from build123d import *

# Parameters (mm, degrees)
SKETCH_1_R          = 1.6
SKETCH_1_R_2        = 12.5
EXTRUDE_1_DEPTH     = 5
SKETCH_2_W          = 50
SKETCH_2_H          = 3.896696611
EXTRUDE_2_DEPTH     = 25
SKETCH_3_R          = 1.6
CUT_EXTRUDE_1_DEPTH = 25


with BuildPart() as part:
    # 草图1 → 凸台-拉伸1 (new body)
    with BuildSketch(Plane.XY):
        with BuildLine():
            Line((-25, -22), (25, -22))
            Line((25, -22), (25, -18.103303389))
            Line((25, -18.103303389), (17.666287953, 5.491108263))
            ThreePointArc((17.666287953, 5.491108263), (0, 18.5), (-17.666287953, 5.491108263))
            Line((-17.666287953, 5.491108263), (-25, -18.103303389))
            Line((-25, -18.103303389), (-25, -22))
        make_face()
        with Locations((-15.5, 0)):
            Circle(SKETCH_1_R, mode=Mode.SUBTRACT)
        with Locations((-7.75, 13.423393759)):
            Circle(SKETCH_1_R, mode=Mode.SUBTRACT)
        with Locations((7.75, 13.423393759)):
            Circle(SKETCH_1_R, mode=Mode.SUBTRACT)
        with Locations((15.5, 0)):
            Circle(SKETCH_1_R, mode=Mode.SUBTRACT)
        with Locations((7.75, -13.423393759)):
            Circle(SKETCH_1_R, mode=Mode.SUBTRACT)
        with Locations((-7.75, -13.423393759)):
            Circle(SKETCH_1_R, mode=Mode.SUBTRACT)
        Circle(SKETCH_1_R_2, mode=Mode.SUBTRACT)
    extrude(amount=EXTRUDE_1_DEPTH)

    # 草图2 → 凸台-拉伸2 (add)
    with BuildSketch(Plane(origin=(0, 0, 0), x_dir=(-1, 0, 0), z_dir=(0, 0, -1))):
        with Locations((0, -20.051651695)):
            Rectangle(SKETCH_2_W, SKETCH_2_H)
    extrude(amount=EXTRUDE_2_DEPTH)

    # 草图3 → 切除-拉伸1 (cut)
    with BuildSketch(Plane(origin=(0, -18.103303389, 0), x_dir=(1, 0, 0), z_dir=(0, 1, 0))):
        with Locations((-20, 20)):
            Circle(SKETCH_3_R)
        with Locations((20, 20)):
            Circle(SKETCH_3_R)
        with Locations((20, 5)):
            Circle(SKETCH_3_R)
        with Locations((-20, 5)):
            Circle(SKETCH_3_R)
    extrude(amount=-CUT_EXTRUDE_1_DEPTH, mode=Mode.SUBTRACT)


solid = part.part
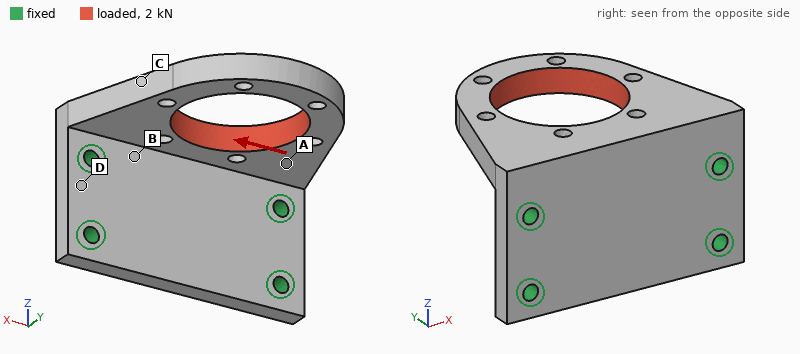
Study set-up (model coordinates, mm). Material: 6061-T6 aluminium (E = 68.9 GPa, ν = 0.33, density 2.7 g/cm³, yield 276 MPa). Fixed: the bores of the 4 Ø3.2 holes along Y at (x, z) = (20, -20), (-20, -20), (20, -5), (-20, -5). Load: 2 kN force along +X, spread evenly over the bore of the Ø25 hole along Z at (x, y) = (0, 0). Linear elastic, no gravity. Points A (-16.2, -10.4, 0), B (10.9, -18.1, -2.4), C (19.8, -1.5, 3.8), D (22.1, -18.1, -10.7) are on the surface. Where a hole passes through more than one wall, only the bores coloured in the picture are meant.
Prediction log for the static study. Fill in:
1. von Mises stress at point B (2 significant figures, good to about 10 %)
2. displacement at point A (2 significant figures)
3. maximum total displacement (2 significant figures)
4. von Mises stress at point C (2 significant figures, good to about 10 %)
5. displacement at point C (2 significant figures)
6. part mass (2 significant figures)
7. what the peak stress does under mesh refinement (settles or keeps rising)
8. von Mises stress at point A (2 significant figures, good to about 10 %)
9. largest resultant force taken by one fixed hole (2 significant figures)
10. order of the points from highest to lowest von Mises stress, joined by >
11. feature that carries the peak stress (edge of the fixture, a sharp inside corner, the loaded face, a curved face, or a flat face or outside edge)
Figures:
43 MPa
0.031 mm
0.11 mm
71 MPa
0.065 mm
26 g
keeps rising
24 MPa
1.4 kN
C > B > A > D
edge of the fixture
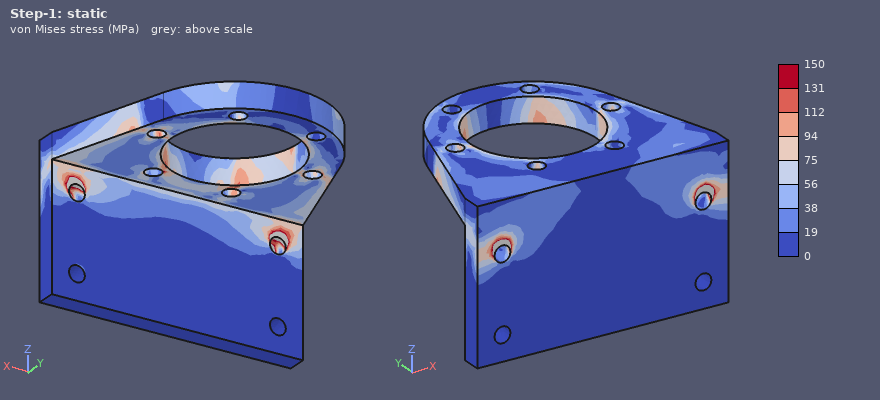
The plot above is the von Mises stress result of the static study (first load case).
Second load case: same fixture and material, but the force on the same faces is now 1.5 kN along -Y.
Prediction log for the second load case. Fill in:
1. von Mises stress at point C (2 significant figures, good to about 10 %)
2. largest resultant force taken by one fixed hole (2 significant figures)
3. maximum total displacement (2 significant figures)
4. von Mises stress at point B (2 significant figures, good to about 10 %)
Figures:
31 MPa
880 N
0.14 mm
32 MPa
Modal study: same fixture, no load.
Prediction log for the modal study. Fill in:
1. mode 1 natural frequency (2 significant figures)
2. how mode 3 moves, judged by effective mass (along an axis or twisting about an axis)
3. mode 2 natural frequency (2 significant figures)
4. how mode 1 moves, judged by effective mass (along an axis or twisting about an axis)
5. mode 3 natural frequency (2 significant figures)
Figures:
2500 Hz
along X
6200 Hz
along Z
9400 Hz
